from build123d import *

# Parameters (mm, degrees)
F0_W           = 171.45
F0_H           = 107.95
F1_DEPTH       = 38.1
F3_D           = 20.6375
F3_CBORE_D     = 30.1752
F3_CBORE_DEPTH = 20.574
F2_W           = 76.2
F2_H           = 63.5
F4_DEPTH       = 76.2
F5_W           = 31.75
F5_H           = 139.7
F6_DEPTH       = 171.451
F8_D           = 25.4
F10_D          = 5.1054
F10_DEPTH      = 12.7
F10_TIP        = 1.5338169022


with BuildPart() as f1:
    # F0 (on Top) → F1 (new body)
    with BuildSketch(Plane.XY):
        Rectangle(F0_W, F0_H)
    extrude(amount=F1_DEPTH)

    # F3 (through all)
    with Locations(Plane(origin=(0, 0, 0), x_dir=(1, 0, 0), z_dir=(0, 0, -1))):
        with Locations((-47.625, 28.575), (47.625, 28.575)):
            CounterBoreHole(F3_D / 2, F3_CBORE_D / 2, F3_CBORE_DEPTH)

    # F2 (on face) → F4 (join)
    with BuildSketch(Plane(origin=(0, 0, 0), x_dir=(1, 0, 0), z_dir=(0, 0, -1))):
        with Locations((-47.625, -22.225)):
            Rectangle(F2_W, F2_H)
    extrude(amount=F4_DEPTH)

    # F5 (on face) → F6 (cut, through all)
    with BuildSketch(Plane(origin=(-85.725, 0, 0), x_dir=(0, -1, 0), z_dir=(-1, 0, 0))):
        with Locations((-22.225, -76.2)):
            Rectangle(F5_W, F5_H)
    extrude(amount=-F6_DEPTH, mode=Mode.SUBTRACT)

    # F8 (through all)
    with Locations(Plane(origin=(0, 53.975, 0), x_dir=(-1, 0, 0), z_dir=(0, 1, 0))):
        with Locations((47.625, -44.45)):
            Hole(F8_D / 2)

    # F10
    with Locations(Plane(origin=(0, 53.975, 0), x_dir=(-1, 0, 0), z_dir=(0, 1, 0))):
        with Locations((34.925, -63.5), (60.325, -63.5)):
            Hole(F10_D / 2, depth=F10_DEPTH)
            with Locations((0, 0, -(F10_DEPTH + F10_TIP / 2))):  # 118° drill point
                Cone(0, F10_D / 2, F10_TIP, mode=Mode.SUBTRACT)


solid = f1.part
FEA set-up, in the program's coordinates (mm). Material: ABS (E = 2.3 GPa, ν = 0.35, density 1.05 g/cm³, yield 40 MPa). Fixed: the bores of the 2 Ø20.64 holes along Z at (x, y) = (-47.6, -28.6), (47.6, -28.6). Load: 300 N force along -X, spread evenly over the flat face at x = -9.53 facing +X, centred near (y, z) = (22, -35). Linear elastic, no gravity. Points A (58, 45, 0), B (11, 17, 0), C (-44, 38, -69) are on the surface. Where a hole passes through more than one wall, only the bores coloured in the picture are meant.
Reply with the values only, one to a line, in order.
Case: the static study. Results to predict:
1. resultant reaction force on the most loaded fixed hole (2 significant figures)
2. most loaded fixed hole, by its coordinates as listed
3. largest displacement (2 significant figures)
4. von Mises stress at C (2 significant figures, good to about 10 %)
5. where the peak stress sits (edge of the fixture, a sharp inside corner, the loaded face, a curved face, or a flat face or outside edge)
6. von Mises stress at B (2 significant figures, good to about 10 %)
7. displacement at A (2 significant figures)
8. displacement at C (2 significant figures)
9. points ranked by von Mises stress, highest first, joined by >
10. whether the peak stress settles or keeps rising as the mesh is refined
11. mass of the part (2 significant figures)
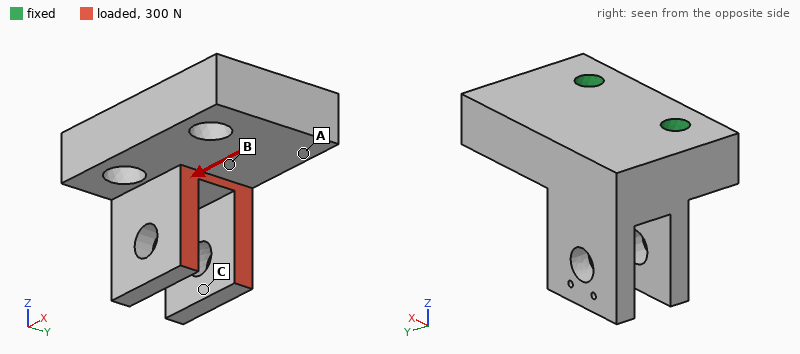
310 N
(47.6, -28.6)
76 µm
0.18 MPa
edge of the fixture
0.30 MPa
15 µm
64 µm
B > C > A
keeps rising
890 g
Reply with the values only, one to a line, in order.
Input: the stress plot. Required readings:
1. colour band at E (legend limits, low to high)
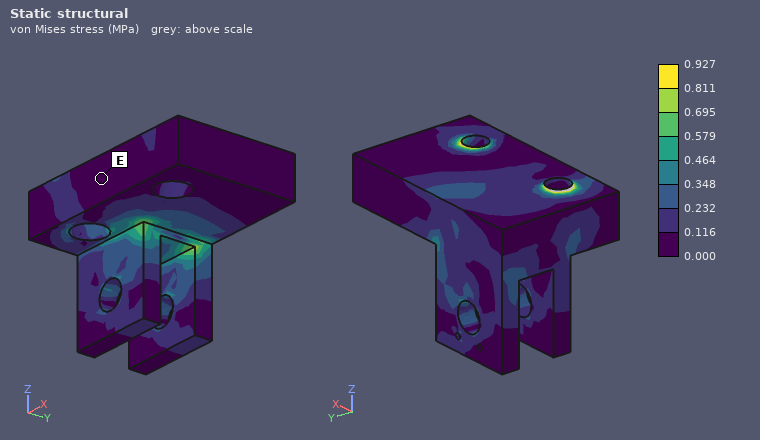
0.000 to 0.116 MPa
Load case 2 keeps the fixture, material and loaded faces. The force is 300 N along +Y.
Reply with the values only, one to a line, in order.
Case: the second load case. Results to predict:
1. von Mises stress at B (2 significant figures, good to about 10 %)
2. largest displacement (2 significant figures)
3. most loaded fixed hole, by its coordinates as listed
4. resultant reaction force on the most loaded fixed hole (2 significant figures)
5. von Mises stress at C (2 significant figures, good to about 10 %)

0.36 MPa
0.39 mm
(-47.6, -28.6)
180 N
0.66 MPa
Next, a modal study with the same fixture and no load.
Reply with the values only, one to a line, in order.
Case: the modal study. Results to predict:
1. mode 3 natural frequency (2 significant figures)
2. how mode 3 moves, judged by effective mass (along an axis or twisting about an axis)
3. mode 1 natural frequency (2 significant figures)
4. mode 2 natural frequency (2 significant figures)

780 Hz
along Z
390 Hz
630 Hz
